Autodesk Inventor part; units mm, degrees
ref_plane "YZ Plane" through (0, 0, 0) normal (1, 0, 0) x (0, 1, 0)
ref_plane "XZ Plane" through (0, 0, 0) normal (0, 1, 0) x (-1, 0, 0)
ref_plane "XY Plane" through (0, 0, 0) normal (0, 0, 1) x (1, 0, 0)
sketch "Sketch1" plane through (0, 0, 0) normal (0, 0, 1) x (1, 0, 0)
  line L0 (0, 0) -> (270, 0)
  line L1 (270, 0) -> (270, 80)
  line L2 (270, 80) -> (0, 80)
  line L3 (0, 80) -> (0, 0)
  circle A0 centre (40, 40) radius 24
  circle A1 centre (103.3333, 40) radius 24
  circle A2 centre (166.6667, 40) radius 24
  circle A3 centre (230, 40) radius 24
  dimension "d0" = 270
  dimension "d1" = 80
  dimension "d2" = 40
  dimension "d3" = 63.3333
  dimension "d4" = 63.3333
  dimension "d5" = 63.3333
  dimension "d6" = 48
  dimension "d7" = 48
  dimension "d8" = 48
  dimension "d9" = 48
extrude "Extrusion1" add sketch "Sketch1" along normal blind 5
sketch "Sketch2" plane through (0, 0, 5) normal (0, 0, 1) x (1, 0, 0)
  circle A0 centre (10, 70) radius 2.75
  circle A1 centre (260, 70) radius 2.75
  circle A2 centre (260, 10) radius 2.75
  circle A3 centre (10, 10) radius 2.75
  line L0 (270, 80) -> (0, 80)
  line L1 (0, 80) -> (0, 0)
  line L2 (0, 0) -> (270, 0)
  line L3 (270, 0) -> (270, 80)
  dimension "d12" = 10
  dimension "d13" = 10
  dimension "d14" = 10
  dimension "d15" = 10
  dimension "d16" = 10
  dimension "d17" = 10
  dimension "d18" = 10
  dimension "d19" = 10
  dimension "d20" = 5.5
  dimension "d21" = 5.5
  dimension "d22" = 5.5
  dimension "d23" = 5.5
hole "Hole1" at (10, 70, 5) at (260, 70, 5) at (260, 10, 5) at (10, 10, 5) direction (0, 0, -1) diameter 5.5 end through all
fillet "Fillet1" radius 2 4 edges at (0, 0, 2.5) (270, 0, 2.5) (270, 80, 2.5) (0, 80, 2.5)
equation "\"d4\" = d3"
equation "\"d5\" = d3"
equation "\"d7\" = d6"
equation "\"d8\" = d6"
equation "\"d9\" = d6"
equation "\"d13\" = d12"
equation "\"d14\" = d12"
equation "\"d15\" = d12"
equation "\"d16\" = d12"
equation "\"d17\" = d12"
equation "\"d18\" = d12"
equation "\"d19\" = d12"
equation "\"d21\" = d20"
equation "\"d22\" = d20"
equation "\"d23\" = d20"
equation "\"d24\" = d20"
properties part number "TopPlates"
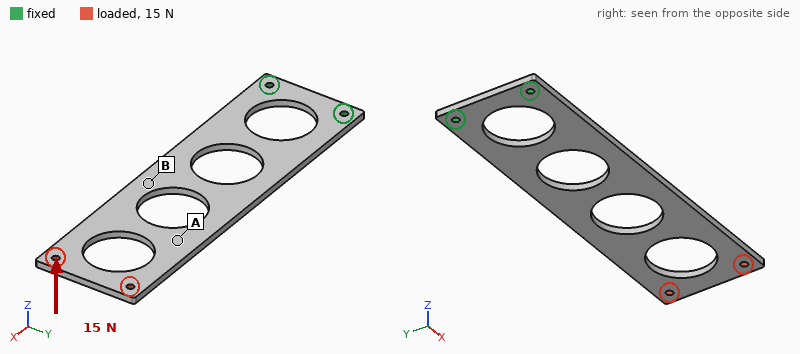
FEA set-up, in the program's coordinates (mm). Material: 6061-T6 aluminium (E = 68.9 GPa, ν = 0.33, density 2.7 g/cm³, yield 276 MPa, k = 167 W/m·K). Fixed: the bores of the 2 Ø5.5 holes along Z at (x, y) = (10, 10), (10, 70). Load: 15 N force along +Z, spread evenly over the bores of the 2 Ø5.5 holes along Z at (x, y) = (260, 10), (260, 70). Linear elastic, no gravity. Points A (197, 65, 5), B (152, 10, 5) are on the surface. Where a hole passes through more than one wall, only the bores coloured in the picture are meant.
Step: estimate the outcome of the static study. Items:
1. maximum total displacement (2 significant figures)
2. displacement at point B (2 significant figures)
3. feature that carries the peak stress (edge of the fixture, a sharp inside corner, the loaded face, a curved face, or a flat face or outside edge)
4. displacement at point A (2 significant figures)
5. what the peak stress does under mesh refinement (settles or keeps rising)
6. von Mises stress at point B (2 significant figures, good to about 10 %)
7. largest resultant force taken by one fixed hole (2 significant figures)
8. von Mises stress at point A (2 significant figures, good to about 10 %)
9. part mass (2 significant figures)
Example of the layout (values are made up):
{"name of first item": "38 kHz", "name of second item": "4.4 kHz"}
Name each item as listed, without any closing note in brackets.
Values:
{"maximum total displacement": "2.8 mm", "displacement at point B": "1.0 mm", "feature that carries the peak stress": "edge of the fixture", "displacement at point A": "1.7 mm", "what the peak stress does under mesh refinement": "keeps rising", "von Mises stress at point B": "9.9 MPa", "largest resultant force taken by one fixed hole": "7.5 N", "von Mises stress at point A": "3.7 MPa", "part mass": "190 g"}
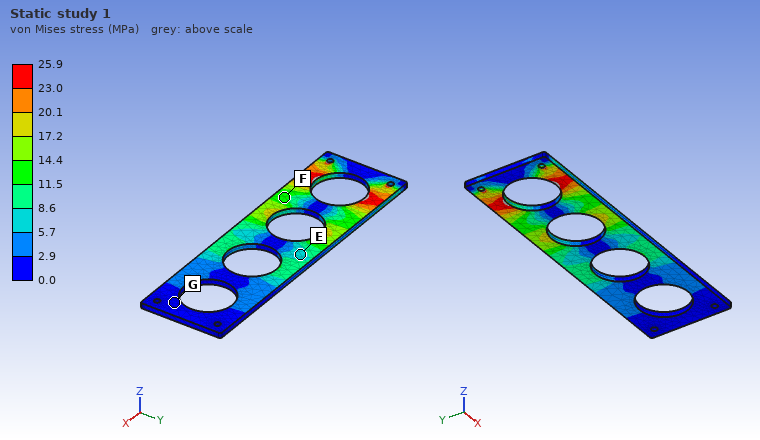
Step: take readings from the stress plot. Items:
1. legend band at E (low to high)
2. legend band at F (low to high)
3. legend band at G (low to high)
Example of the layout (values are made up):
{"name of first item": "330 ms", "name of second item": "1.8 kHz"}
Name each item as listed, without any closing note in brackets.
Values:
{"legend band at E": "5.7 to 8.6 MPa", "legend band at F": "11.5 to 14.4 MPa", "legend band at G": "0.0 to 2.9 MPa"}
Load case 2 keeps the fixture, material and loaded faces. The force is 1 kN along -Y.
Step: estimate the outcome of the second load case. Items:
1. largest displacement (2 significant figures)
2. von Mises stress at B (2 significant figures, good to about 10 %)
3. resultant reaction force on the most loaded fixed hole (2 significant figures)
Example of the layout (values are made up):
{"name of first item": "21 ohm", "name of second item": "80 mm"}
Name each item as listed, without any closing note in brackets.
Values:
{"largest displacement": "0.69 mm", "von Mises stress at B": "21 MPa", "resultant reaction force on the most loaded fixed hole": "3.9 kN"}
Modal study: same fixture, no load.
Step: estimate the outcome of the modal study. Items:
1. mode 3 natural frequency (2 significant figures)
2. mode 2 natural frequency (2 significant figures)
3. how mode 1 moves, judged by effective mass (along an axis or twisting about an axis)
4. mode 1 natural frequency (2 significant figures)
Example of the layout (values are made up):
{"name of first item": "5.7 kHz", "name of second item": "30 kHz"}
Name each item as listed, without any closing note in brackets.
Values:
{"mode 3 natural frequency": "330 Hz", "mode 2 natural frequency": "320 Hz", "how mode 1 moves, judged by effective mass": "along Z", "mode 1 natural frequency": "52 Hz"}
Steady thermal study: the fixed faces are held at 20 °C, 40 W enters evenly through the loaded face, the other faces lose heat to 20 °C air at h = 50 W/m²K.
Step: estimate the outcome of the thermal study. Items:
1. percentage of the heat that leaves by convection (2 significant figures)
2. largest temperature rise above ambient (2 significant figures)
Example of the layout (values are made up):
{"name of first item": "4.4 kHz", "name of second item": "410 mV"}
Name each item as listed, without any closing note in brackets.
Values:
{"percentage of the heat that leaves by convection": "94 %", "largest temperature rise above ambient": "75 K"}
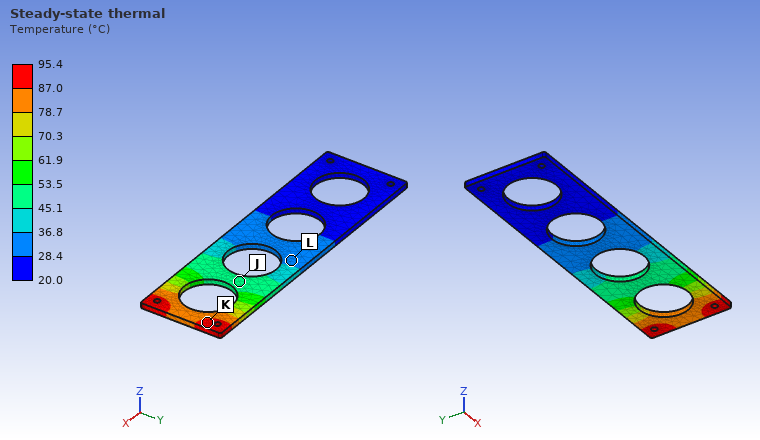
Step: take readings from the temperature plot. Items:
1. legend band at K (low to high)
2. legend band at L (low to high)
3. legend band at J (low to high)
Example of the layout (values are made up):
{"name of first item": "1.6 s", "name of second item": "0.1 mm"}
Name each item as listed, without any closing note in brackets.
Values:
{"legend band at K": "87.0 to 95.4 °C", "legend band at L": "28.4 to 36.8 °C", "legend band at J": "45.1 to 53.5 °C"}
